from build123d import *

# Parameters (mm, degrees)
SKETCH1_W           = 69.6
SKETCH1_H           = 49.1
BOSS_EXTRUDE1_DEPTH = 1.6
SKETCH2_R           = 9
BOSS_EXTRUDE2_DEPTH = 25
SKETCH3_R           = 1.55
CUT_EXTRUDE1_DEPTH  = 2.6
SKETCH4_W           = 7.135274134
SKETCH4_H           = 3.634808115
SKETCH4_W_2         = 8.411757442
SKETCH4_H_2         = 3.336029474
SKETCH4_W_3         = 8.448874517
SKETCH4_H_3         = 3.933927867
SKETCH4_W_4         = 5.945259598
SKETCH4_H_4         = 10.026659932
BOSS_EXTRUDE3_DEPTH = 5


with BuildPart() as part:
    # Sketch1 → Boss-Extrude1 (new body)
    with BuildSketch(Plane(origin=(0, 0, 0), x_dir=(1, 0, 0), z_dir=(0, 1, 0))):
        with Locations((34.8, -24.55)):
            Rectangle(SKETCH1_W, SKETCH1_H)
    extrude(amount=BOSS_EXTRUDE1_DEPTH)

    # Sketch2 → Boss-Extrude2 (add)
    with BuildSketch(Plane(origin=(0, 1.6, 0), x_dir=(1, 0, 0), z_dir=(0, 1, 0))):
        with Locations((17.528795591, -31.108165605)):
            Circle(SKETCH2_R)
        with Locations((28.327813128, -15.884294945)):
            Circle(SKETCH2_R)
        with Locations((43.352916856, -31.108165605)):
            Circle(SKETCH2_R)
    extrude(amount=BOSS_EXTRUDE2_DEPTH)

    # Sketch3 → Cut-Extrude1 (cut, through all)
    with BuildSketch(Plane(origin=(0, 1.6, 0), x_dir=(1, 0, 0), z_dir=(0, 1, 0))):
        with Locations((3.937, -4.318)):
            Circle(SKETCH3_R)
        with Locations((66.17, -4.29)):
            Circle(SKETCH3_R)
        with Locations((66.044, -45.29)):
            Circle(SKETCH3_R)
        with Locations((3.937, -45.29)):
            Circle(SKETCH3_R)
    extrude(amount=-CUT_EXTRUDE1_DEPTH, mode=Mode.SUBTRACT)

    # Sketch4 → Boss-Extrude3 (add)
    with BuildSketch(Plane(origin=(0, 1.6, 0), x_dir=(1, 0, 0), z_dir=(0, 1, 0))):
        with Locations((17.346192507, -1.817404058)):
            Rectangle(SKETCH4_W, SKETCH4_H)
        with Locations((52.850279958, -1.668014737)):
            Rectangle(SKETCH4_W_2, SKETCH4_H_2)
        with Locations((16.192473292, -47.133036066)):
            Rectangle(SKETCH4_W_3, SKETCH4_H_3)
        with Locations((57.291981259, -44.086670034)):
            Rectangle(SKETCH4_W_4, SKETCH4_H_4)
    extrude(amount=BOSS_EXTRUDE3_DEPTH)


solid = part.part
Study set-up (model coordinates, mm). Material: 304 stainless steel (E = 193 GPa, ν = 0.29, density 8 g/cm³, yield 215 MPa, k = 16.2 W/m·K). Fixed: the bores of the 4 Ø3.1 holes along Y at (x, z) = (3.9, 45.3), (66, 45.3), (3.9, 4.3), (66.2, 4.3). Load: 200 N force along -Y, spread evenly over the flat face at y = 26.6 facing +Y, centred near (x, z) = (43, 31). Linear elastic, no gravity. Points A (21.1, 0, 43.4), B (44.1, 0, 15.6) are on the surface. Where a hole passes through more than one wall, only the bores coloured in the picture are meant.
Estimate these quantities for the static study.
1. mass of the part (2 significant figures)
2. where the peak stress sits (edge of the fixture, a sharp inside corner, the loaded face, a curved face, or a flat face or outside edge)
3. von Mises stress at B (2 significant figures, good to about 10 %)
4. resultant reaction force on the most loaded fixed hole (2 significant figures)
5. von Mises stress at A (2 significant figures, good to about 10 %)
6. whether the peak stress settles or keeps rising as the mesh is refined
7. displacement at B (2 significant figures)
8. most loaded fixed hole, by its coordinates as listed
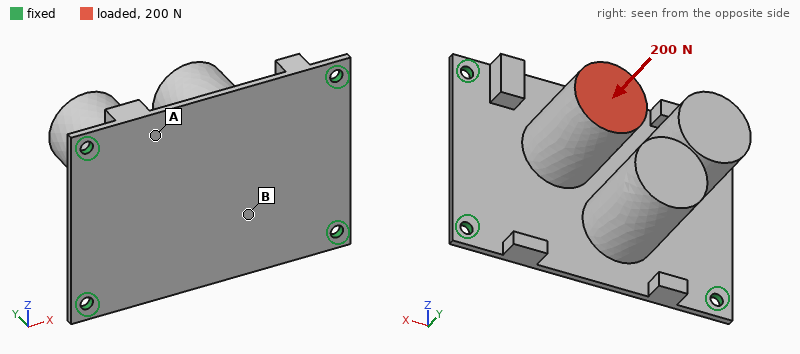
200 g
edge of the fixture
30 MPa
92 N
10 MPa
keeps rising
48 µm
(66, 45.3)
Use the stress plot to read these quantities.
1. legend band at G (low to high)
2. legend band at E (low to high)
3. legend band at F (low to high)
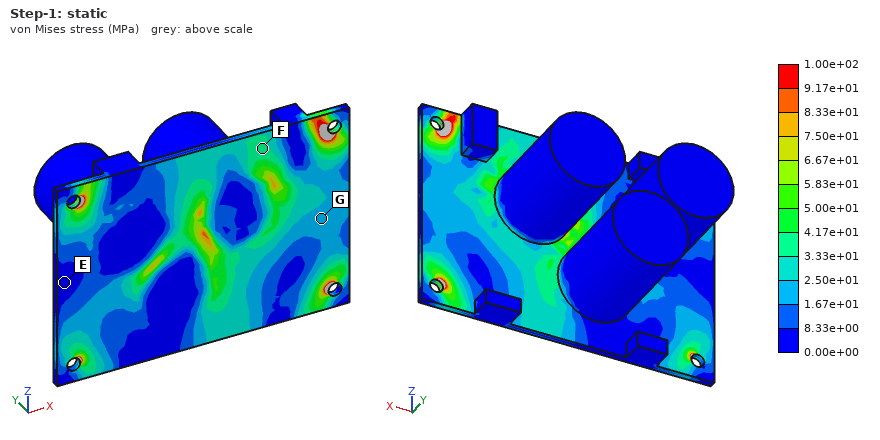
1.67e+01 to 2.50e+01 MPa
0.00e+00 to 8.33e+00 MPa
3.33e+01 to 4.17e+01 MPa
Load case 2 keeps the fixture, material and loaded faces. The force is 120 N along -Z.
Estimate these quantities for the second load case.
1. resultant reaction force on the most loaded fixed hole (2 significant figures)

62 N
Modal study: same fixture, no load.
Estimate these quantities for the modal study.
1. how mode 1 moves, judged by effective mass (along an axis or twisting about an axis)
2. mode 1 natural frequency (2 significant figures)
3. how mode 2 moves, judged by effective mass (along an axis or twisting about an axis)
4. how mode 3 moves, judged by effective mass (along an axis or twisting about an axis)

along Y
750 Hz
along Z
along X
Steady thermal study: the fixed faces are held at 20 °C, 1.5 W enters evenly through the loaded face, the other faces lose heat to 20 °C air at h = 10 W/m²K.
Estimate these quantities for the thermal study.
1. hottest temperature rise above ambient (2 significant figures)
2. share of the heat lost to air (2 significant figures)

21 K
52 %
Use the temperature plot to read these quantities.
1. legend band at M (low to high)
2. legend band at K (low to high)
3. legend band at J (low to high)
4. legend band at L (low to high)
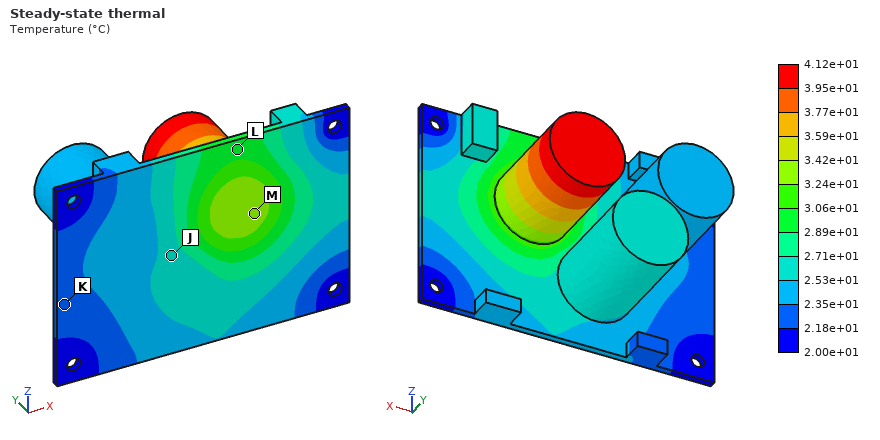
3.24e+01 to 3.42e+01 °C
2.18e+01 to 2.35e+01 °C
2.53e+01 to 2.71e+01 °C
2.89e+01 to 3.06e+01 °C
